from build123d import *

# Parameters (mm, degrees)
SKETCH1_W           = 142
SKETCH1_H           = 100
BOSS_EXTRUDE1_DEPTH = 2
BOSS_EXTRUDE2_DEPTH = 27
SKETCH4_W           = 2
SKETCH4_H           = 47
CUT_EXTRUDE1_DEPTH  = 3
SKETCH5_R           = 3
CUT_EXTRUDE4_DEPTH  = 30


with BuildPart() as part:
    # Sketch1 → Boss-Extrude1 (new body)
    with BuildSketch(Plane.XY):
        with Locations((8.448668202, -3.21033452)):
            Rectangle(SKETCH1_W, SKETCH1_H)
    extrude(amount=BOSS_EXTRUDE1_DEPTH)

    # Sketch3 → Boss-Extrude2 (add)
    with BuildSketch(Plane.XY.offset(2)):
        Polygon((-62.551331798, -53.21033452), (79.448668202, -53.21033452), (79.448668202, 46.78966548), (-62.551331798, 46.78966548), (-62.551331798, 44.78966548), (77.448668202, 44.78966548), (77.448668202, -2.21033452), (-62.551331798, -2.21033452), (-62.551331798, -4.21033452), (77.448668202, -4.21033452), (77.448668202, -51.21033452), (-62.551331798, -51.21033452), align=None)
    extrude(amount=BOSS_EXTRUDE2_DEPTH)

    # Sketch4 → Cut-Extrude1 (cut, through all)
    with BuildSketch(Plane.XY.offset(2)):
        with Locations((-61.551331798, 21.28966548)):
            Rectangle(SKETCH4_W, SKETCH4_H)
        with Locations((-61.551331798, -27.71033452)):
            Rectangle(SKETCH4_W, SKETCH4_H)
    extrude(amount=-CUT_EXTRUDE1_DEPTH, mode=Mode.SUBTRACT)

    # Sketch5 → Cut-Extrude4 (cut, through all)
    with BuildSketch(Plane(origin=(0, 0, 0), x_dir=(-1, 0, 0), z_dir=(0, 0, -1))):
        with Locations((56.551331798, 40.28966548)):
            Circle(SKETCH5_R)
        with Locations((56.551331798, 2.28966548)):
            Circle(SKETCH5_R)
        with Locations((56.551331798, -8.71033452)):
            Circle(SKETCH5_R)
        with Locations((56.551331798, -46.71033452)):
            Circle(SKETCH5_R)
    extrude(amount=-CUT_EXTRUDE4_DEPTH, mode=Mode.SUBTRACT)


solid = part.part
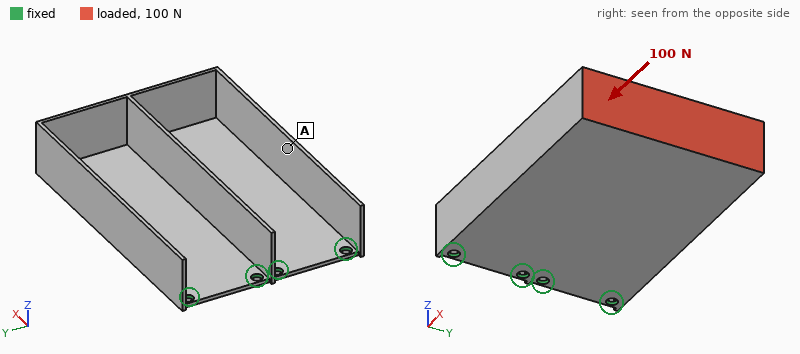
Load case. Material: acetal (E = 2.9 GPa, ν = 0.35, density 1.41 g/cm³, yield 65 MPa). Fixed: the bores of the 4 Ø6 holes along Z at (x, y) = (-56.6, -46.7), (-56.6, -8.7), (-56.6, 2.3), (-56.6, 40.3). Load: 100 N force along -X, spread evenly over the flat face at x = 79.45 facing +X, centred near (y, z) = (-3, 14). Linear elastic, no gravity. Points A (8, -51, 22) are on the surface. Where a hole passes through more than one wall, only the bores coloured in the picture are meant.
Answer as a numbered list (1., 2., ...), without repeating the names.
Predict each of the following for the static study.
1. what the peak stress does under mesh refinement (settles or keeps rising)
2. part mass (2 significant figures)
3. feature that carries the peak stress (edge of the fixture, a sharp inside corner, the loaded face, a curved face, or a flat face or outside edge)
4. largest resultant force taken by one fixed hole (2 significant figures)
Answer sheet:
1. keeps rising
2. 79 g
3. edge of the fixture
4. 26 N
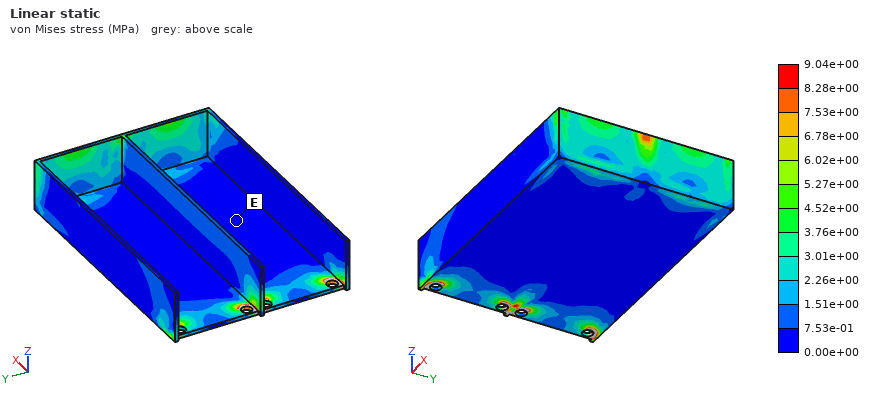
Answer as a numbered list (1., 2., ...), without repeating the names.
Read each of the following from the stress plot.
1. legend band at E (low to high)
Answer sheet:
1. 0.00e+00 to 7.53e-01 MPa
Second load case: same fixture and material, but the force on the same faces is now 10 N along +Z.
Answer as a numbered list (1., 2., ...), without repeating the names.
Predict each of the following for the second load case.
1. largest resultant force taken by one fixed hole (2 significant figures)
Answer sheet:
1. 5.9 N
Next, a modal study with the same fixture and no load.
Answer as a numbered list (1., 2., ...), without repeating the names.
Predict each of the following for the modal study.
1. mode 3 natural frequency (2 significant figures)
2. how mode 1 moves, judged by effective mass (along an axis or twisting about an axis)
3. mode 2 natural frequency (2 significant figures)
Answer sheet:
1. 390 Hz
2. along Z
3. 82 Hz
